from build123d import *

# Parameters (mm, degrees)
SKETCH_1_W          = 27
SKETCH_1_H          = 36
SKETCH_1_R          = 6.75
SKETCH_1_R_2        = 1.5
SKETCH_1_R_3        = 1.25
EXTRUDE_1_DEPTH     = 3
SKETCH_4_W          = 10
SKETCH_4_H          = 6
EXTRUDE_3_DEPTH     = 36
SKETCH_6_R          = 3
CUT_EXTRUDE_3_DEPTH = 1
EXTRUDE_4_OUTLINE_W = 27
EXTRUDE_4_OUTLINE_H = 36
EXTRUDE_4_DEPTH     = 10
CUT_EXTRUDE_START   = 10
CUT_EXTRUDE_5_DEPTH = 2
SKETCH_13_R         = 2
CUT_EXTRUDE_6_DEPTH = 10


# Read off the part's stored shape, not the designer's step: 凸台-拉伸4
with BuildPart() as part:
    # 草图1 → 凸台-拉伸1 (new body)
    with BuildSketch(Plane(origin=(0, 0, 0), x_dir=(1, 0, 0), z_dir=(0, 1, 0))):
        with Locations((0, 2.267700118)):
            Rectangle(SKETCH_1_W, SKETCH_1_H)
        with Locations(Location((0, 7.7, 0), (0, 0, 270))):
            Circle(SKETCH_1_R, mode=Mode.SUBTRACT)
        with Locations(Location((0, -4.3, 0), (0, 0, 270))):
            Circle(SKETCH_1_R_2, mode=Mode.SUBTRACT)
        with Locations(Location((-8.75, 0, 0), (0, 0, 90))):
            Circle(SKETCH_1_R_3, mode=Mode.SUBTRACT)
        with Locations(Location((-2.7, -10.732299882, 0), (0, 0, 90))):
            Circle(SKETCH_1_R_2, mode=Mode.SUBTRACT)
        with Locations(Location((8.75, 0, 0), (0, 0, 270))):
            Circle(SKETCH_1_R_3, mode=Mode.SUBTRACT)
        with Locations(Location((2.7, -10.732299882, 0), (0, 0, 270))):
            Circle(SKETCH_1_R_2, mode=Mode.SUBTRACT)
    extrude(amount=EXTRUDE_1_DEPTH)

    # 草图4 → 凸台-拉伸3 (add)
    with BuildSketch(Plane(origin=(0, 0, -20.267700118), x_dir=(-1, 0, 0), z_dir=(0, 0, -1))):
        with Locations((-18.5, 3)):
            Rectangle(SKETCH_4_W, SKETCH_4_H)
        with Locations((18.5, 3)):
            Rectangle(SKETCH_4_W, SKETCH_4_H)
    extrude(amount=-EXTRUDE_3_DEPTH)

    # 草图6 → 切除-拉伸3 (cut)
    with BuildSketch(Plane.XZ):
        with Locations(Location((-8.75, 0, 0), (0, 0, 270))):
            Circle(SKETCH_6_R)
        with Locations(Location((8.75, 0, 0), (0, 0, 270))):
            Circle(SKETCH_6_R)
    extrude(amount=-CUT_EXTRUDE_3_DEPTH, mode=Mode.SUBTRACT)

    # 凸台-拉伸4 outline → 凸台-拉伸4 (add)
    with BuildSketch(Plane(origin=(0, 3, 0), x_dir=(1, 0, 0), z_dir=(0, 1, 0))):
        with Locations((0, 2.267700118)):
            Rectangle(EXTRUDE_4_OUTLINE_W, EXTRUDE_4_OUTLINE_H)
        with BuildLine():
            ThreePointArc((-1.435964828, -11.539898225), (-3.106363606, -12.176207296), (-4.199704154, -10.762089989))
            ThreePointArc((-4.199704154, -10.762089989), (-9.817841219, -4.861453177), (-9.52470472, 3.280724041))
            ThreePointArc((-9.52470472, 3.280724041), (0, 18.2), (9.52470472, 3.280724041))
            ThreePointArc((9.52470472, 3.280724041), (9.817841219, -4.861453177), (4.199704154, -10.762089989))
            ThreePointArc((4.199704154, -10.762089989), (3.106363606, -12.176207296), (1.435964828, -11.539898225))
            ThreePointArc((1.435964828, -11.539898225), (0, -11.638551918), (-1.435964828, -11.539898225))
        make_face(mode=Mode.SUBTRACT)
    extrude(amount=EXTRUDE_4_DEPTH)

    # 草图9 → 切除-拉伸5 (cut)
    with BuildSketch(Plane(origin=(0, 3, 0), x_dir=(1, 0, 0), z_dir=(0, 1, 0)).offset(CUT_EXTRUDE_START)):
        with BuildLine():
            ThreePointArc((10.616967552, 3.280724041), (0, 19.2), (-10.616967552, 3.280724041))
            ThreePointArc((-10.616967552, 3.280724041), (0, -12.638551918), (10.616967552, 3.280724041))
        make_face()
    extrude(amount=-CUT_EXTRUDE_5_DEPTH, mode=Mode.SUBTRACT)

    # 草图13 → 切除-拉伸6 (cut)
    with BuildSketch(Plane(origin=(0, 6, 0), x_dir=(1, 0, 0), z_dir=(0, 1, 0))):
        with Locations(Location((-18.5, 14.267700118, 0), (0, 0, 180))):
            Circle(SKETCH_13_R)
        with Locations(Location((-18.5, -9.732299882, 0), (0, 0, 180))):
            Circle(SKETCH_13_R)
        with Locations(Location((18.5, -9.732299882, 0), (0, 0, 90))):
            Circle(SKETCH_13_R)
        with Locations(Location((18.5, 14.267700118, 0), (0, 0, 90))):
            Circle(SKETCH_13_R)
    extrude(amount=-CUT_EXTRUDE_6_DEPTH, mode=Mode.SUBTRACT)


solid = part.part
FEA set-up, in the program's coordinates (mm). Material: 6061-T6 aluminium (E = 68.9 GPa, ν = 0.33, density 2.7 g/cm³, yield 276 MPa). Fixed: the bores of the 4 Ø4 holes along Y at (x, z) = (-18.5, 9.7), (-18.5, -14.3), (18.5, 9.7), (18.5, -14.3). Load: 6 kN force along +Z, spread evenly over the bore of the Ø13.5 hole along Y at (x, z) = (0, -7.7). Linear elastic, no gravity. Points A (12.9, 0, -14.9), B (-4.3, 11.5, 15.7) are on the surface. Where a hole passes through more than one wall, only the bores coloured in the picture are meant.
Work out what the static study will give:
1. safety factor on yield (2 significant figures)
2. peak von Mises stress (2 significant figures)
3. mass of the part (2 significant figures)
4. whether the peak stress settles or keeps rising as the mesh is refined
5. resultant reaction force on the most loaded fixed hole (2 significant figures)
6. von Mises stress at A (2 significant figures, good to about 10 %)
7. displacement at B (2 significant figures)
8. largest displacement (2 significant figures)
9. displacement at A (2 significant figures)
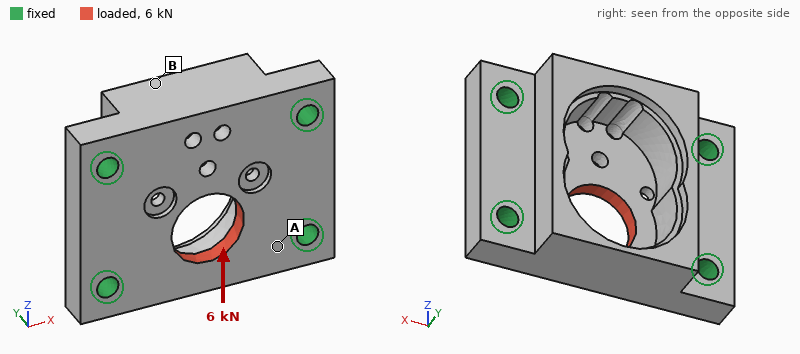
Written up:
1.8
150 MPa
29 g
settles
1.7 kN
36 MPa
4.5 µm
28 µm
5.7 µm
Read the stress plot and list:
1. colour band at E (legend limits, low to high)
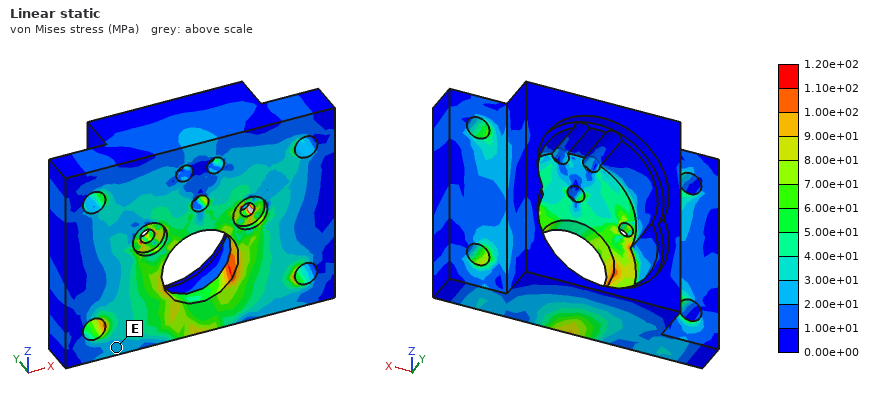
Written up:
2.00e+01 to 3.00e+01 MPa
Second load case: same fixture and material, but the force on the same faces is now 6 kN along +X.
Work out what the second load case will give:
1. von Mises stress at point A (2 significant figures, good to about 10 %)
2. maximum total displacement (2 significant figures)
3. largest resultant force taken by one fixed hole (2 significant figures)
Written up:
43 MPa
13 µm
2.1 kN
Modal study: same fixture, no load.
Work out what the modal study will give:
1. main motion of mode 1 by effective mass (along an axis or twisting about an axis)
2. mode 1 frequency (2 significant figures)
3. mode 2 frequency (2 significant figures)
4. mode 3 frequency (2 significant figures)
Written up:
along Y
21 kHz
22 kHz
31 kHz
